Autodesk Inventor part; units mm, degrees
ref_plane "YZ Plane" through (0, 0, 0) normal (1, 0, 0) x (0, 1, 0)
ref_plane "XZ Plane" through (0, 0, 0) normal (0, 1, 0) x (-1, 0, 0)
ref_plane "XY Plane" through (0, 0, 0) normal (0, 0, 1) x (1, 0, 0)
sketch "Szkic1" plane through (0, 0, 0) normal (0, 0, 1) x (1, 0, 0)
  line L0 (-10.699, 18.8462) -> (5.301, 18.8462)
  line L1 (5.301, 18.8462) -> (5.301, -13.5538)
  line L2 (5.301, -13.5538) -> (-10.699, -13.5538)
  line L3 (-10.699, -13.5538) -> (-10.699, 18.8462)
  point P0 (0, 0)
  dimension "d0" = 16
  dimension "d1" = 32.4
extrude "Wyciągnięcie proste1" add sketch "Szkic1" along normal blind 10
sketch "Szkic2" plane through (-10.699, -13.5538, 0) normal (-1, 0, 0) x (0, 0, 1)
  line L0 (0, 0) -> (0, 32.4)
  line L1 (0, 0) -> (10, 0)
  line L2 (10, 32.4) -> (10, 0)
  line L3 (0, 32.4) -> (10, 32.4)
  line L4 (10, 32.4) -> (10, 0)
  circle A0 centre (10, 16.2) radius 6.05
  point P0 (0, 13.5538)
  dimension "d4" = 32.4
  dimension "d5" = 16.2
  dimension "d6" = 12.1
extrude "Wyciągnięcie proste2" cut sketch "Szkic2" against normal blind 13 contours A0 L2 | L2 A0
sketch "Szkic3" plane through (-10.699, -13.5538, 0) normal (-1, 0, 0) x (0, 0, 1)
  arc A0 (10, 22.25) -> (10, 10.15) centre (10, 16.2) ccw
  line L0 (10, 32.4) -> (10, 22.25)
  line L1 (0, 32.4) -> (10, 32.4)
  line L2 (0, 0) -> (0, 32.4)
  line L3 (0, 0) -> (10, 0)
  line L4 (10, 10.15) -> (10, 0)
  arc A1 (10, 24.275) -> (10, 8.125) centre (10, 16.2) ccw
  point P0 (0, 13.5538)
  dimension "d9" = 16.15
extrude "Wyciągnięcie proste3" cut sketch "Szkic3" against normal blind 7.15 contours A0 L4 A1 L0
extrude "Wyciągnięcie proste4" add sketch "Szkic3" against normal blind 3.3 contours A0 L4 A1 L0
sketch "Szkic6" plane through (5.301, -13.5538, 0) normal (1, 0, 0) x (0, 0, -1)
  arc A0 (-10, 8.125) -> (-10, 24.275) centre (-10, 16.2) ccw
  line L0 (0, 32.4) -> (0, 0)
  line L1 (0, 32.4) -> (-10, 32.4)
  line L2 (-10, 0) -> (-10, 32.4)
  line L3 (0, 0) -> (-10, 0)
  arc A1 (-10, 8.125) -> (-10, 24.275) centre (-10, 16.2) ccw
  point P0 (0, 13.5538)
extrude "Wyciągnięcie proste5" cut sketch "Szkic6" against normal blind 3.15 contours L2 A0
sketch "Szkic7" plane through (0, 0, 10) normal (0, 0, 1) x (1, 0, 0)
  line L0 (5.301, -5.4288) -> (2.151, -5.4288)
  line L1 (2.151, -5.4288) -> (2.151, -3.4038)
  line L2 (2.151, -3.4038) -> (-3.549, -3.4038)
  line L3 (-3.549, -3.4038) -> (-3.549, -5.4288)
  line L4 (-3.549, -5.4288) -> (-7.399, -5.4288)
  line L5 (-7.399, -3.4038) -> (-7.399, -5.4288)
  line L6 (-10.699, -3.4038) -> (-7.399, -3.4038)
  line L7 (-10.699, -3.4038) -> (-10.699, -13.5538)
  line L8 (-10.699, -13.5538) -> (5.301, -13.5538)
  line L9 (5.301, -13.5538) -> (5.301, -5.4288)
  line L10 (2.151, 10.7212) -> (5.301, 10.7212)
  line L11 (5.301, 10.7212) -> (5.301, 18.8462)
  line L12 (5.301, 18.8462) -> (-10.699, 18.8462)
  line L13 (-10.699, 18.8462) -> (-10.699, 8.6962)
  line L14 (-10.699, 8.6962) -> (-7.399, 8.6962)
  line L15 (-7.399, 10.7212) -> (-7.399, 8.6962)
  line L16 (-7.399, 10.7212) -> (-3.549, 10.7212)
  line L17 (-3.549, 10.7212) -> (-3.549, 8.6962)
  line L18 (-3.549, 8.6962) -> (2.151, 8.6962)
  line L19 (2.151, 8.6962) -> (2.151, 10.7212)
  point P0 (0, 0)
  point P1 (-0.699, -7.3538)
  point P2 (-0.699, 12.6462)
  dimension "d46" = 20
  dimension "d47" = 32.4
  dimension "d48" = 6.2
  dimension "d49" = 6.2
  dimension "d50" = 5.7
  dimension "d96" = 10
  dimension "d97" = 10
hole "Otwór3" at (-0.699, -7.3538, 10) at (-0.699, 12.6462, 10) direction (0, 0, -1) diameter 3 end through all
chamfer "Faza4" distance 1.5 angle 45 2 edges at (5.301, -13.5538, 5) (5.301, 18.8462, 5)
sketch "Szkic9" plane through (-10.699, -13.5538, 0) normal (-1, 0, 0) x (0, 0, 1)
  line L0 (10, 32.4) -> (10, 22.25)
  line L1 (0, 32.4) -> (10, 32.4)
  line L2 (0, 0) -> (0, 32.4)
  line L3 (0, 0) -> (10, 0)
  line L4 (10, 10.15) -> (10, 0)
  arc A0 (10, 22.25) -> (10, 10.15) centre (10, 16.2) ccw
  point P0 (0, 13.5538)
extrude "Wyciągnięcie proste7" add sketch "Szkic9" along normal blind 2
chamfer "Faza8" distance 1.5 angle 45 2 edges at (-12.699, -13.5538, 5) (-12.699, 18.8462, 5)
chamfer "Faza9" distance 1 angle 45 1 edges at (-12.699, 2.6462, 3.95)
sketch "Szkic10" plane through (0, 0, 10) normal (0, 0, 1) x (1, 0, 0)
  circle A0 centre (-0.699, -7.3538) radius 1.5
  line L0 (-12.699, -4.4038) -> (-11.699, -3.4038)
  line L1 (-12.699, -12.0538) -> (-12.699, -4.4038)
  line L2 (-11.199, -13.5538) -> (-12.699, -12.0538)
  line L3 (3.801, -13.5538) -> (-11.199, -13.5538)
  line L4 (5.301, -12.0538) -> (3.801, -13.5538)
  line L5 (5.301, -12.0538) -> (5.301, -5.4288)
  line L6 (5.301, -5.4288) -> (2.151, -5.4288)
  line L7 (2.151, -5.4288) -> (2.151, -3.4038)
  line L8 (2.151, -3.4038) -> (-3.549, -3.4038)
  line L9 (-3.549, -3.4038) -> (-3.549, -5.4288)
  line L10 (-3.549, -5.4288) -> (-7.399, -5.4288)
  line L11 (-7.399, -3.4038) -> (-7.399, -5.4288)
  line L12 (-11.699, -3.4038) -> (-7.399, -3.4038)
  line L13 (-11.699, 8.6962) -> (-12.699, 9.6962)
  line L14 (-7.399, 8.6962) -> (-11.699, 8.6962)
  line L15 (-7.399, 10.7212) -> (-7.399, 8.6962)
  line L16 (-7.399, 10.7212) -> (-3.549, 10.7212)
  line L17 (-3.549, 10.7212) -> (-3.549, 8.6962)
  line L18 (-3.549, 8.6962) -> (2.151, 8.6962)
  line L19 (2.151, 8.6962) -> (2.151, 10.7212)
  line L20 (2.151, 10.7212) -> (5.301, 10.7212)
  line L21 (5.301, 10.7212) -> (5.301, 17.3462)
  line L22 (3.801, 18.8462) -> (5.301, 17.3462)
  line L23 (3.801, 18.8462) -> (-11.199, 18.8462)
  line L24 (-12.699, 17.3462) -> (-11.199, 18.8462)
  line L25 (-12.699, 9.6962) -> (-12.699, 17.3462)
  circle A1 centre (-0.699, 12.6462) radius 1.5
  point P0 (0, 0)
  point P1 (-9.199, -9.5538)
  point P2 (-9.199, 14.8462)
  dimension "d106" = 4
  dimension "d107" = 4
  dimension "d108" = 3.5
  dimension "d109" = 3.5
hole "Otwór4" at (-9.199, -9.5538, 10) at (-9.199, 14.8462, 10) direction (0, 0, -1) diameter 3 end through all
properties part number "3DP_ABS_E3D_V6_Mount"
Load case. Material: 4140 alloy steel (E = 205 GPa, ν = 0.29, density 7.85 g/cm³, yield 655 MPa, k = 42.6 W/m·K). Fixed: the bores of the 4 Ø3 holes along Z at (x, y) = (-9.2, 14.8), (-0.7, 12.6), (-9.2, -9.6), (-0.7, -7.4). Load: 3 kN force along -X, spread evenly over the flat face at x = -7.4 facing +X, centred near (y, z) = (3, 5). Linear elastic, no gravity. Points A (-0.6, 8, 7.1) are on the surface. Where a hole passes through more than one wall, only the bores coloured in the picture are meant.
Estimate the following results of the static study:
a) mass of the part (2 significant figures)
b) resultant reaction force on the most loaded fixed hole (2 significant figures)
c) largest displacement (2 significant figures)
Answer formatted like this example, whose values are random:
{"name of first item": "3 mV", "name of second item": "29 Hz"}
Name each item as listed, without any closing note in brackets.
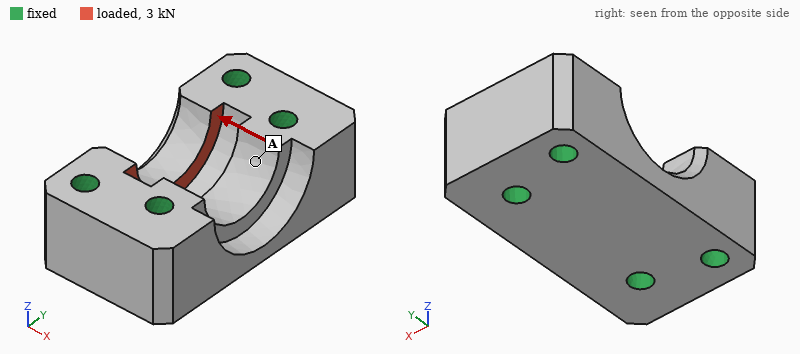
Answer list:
{"mass of the part": "33 g", "resultant reaction force on the most loaded fixed hole": "1.1 kN", "largest displacement": "3.9 µm"}
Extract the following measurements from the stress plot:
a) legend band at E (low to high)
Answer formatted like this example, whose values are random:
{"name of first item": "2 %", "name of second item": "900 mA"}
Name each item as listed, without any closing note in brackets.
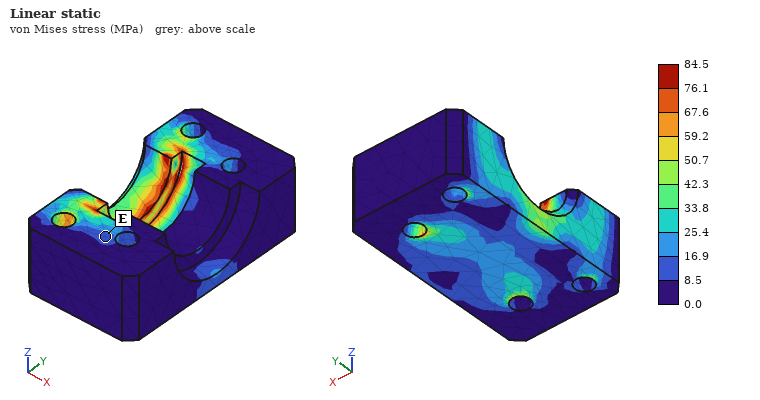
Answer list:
{"legend band at E": "8.5 to 16.9 MPa"}
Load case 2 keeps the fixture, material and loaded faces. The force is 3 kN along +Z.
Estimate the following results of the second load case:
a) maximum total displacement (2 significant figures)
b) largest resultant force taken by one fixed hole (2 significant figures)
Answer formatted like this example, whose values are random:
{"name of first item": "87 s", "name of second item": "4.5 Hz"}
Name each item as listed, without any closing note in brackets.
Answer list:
{"maximum total displacement": "5.5 µm", "largest resultant force taken by one fixed hole": "1.1 kN"}
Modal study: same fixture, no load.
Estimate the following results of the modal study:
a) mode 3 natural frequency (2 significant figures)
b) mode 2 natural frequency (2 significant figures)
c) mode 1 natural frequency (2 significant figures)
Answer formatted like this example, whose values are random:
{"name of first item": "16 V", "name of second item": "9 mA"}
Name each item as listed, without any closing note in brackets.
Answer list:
{"mode 3 natural frequency": "83 kHz", "mode 2 natural frequency": "73 kHz", "mode 1 natural frequency": "69 kHz"}
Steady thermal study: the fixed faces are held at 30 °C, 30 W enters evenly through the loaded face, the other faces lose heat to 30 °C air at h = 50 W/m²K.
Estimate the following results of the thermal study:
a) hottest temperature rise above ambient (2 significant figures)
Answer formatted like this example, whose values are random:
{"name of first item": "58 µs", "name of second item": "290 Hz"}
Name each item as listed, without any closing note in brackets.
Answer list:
{"hottest temperature rise above ambient": "53 K"}
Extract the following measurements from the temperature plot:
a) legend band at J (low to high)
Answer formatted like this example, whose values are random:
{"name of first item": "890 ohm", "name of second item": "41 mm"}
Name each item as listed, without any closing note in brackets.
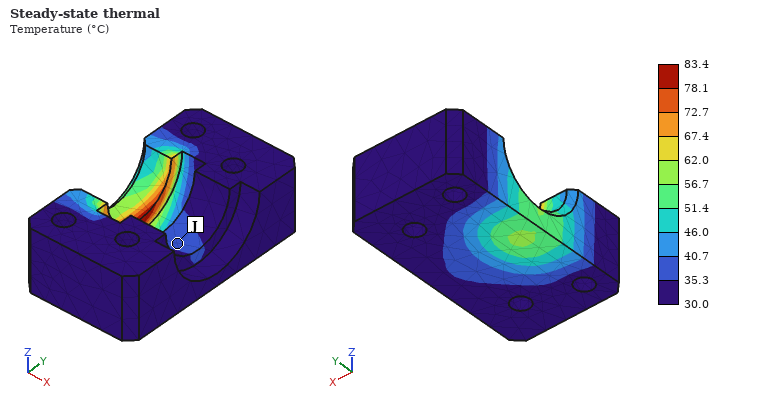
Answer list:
{"legend band at J": "35.3 to 40.7 °C"}
